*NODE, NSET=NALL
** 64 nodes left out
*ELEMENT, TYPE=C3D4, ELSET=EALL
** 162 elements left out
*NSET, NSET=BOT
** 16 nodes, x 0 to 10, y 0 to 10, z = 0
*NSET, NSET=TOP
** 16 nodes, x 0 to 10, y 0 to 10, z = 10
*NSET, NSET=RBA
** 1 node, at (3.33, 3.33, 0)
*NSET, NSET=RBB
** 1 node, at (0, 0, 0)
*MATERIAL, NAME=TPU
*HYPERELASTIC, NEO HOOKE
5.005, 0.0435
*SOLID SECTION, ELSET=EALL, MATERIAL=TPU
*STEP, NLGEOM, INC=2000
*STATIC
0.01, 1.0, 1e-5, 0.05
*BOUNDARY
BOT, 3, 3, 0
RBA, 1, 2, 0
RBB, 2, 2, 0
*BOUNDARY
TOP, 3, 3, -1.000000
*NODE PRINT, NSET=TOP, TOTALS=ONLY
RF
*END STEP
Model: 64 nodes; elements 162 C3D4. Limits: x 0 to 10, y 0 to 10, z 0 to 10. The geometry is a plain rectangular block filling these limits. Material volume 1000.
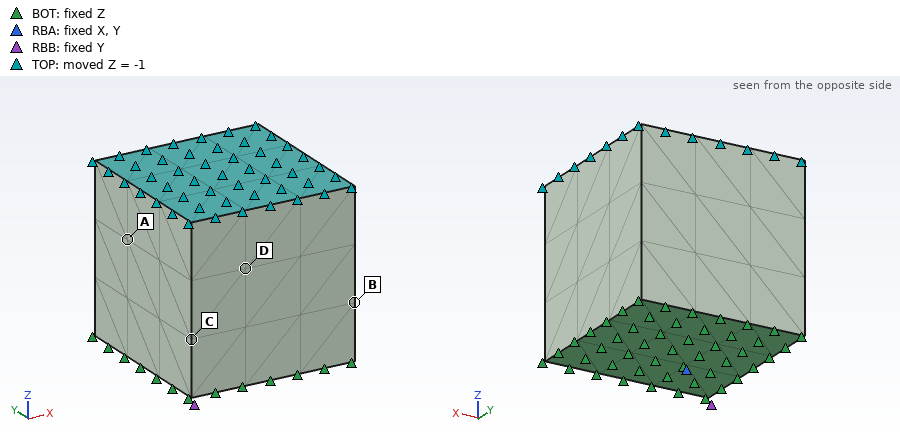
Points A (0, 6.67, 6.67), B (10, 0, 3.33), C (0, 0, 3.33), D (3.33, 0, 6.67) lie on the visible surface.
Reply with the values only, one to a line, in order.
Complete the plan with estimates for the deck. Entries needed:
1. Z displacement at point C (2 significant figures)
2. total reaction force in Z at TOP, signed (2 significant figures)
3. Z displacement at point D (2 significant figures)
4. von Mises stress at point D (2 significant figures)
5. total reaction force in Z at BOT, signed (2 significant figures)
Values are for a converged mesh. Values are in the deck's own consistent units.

-0.33
-310
-0.67
2.9
310
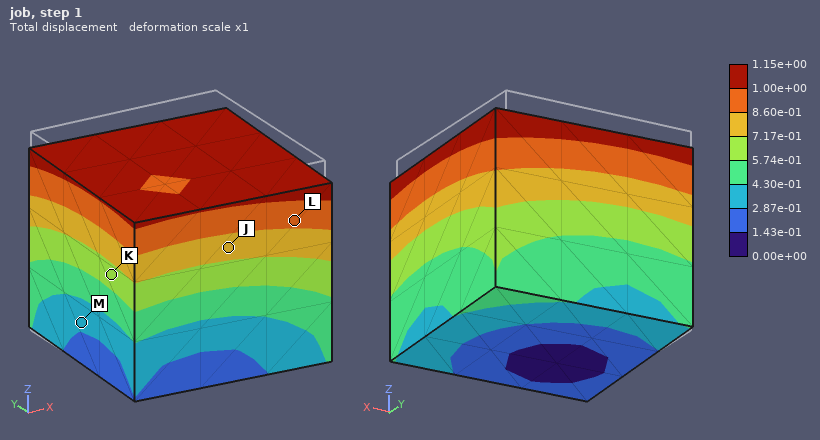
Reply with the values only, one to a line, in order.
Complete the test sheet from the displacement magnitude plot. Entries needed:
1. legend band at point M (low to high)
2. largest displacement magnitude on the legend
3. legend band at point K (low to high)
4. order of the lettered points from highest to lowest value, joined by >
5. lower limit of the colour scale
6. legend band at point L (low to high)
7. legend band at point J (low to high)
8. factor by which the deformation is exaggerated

2.87e-01 to 4.30e-01
1.15e+00
5.74e-01 to 7.17e-01
L > J > K > M
0.00e+00
8.60e-01 to 1.00e+00
7.17e-01 to 8.60e-01
1
